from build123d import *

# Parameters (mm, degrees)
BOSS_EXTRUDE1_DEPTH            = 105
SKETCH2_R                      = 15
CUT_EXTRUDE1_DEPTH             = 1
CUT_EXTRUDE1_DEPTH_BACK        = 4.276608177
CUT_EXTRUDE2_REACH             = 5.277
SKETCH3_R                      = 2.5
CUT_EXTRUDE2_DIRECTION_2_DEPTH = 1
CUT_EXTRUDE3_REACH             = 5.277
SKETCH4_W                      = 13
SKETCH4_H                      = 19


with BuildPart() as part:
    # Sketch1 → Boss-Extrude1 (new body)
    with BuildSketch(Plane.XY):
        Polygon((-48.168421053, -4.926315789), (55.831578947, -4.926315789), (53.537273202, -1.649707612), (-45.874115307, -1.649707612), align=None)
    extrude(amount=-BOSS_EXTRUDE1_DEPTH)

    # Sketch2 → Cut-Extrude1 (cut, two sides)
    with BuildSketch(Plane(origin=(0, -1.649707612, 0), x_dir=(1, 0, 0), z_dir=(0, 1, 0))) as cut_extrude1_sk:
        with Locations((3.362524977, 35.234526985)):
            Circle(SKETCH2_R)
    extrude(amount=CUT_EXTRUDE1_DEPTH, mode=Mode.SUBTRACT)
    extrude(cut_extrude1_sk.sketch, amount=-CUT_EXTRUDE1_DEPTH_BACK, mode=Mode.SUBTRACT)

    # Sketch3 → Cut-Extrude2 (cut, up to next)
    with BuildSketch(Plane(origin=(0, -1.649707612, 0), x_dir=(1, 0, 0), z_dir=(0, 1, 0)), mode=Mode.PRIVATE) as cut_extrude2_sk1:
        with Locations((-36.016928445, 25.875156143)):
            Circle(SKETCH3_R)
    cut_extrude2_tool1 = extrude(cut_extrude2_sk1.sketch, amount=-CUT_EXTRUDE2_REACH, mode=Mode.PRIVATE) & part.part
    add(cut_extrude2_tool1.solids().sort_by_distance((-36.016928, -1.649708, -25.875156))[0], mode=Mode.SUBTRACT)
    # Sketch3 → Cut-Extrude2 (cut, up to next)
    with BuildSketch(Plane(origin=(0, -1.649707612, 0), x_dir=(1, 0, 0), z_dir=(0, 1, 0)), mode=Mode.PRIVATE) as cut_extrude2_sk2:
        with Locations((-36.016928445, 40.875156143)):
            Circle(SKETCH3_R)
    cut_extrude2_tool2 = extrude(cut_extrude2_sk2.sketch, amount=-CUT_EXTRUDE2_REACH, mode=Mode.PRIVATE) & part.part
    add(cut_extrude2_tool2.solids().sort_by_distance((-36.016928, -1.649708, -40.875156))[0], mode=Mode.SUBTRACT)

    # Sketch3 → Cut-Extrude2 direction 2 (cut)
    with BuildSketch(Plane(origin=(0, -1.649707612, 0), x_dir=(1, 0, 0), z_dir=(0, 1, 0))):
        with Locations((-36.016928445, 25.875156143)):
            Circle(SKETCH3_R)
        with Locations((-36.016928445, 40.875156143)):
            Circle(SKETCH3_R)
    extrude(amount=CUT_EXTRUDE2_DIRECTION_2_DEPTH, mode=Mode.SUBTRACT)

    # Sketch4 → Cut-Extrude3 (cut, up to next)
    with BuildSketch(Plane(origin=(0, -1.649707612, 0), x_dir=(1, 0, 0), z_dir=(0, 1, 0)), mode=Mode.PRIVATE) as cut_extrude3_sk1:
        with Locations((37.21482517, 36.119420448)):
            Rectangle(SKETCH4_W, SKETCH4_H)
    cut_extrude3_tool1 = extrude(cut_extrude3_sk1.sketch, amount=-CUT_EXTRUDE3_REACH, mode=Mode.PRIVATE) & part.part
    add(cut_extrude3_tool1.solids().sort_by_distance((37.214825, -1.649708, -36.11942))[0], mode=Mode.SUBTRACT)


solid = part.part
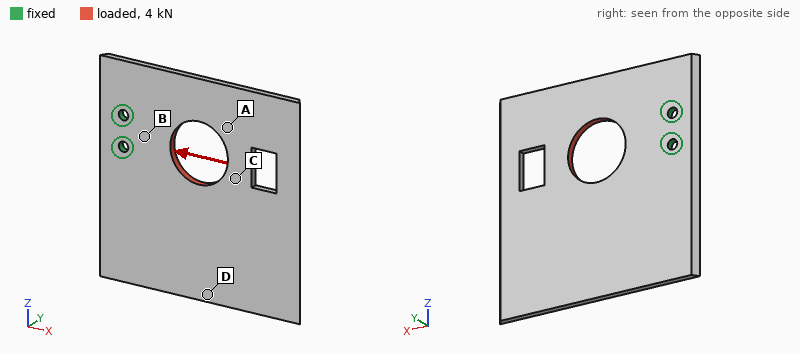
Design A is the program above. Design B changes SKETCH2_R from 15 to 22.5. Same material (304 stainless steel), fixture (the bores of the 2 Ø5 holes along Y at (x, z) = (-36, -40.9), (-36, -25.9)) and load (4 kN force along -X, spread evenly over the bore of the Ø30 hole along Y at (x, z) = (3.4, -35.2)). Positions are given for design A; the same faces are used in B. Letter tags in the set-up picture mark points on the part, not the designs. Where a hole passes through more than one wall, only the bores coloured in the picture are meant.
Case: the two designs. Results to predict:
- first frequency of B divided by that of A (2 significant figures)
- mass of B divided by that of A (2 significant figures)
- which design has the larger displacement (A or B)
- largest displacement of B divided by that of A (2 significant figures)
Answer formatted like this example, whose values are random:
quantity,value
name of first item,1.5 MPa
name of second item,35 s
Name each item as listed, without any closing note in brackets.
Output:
quantity,value
first frequency of B divided by that of A,0.90
mass of B divided by that of A,0.91
which design has the larger displacement,B
largest displacement of B divided by that of A,1.9
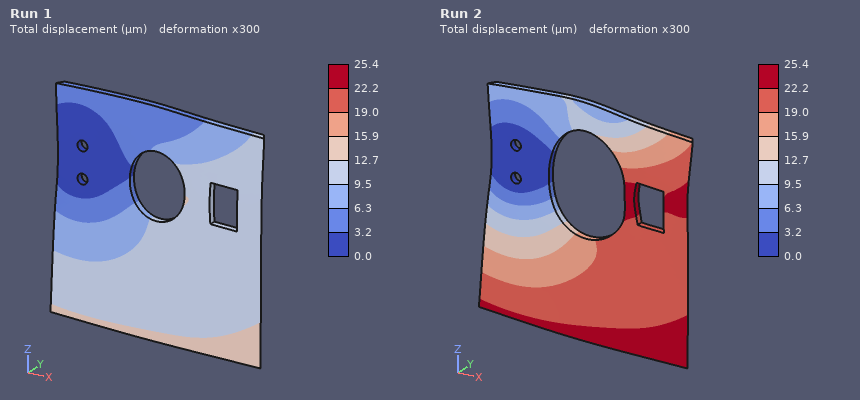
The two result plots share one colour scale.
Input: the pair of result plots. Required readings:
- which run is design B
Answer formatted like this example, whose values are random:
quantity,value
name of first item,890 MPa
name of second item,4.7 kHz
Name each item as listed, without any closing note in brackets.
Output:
quantity,value
which run is design B,Run 2
